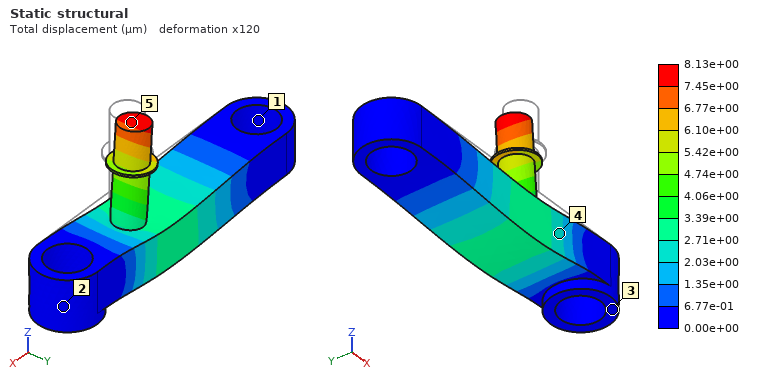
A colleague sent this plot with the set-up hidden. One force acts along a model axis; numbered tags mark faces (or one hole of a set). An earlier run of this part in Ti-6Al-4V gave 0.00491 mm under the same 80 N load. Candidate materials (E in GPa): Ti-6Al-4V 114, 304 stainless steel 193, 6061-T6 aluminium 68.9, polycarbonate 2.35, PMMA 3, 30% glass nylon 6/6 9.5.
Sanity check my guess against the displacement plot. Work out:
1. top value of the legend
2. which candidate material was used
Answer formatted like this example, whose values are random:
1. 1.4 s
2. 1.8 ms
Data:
1. 8.13e+00 µm
2. 6061-T6 aluminium
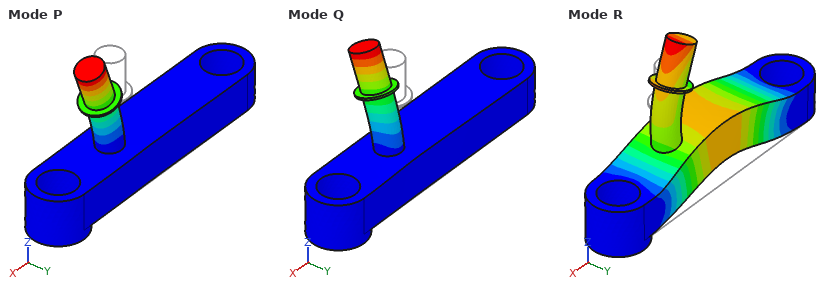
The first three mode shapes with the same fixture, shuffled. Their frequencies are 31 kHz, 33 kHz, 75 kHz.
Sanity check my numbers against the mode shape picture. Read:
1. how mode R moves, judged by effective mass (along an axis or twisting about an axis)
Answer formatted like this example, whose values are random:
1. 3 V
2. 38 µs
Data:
1. along Z
